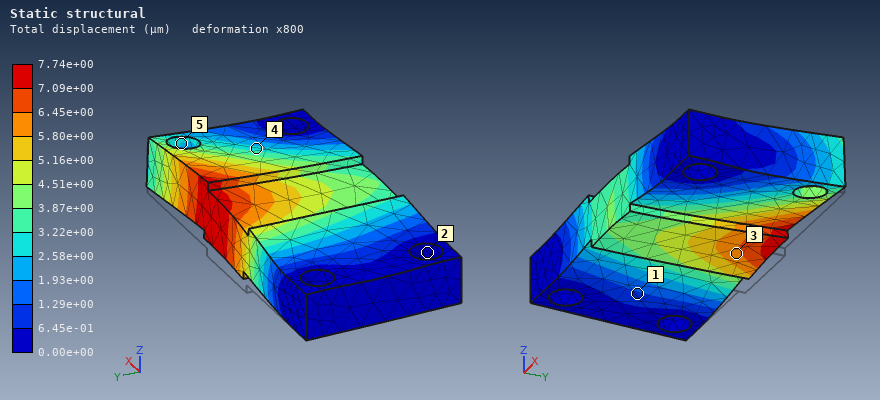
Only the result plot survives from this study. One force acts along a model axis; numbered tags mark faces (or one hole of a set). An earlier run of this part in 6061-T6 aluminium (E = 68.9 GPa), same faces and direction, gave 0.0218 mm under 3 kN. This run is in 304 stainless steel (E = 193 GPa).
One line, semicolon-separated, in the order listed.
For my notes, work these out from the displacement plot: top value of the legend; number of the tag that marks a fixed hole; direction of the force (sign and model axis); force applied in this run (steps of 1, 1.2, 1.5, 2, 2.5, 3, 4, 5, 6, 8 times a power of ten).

7.74e+00 µm; 2; +Z; 3 kN
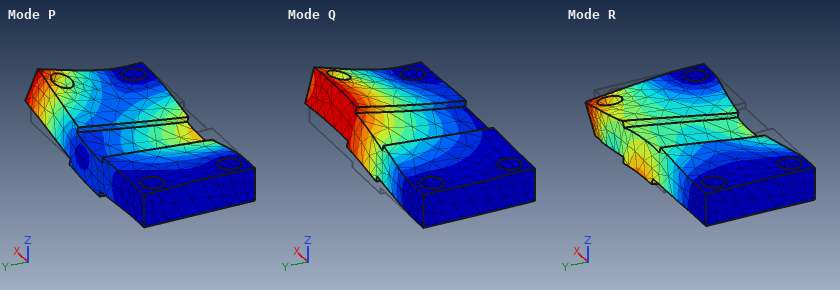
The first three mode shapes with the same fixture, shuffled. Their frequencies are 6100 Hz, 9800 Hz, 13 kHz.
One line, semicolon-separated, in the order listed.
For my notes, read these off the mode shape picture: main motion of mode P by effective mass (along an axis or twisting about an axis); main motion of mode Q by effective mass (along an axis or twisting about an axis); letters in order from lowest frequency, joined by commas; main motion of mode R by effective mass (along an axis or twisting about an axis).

along Z; along Z; Q, P, R; along Y
